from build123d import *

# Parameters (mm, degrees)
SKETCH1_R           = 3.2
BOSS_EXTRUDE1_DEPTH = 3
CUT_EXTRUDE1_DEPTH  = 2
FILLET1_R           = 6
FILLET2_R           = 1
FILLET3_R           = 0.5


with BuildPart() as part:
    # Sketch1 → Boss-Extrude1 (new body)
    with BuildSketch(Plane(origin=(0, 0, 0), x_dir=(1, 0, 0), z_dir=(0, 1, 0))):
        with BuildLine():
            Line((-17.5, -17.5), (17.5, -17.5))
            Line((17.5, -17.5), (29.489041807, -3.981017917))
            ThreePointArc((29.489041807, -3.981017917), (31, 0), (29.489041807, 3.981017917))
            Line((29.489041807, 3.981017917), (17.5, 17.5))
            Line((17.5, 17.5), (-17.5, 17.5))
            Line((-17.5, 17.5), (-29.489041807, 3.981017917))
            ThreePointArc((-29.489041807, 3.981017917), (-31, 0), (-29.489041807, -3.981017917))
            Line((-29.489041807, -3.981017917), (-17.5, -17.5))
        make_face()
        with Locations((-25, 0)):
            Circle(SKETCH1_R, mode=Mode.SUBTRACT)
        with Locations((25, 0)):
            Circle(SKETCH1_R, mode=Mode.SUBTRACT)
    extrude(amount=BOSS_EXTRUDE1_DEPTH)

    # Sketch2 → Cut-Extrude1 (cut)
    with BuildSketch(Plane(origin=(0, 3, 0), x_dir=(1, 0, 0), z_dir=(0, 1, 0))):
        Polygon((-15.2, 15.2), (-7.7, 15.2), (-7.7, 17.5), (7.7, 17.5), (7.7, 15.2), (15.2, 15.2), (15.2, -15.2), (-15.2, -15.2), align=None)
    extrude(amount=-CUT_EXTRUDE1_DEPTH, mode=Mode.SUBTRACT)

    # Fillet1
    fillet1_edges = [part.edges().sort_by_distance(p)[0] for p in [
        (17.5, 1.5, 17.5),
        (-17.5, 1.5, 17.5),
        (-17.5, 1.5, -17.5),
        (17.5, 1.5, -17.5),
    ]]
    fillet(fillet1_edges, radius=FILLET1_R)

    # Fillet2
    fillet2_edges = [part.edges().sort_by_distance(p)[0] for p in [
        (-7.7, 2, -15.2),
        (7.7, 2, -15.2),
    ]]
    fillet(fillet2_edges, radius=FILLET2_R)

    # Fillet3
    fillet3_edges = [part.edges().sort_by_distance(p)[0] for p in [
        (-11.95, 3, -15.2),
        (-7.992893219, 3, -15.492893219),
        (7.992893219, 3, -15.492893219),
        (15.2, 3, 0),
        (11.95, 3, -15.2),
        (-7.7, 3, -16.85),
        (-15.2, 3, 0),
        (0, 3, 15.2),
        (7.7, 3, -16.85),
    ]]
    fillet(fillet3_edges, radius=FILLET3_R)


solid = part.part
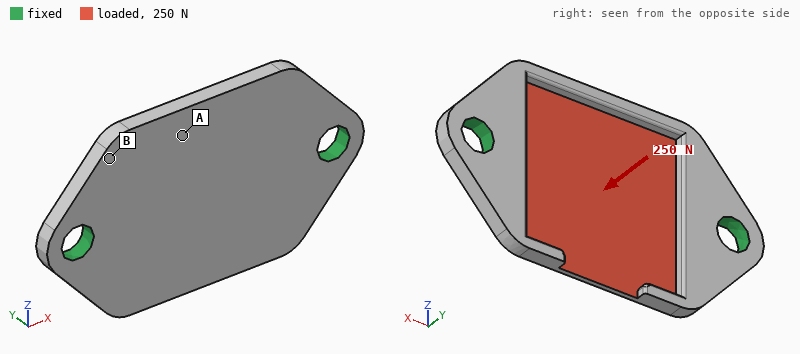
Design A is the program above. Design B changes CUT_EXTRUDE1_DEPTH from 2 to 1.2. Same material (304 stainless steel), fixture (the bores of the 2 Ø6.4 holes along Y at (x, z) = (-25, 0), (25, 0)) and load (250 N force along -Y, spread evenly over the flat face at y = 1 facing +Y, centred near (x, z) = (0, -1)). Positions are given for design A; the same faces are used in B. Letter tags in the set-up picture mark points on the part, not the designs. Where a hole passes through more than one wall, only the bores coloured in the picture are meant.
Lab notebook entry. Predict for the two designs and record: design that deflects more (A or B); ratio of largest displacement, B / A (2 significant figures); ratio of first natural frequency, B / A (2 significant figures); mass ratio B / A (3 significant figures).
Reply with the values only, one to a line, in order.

A
0.56
0.99
1.24
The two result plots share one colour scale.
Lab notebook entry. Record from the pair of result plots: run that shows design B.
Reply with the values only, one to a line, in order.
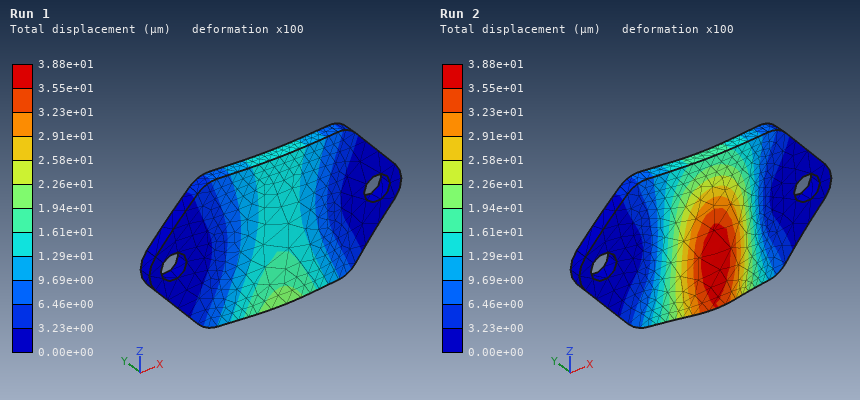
Run 1
